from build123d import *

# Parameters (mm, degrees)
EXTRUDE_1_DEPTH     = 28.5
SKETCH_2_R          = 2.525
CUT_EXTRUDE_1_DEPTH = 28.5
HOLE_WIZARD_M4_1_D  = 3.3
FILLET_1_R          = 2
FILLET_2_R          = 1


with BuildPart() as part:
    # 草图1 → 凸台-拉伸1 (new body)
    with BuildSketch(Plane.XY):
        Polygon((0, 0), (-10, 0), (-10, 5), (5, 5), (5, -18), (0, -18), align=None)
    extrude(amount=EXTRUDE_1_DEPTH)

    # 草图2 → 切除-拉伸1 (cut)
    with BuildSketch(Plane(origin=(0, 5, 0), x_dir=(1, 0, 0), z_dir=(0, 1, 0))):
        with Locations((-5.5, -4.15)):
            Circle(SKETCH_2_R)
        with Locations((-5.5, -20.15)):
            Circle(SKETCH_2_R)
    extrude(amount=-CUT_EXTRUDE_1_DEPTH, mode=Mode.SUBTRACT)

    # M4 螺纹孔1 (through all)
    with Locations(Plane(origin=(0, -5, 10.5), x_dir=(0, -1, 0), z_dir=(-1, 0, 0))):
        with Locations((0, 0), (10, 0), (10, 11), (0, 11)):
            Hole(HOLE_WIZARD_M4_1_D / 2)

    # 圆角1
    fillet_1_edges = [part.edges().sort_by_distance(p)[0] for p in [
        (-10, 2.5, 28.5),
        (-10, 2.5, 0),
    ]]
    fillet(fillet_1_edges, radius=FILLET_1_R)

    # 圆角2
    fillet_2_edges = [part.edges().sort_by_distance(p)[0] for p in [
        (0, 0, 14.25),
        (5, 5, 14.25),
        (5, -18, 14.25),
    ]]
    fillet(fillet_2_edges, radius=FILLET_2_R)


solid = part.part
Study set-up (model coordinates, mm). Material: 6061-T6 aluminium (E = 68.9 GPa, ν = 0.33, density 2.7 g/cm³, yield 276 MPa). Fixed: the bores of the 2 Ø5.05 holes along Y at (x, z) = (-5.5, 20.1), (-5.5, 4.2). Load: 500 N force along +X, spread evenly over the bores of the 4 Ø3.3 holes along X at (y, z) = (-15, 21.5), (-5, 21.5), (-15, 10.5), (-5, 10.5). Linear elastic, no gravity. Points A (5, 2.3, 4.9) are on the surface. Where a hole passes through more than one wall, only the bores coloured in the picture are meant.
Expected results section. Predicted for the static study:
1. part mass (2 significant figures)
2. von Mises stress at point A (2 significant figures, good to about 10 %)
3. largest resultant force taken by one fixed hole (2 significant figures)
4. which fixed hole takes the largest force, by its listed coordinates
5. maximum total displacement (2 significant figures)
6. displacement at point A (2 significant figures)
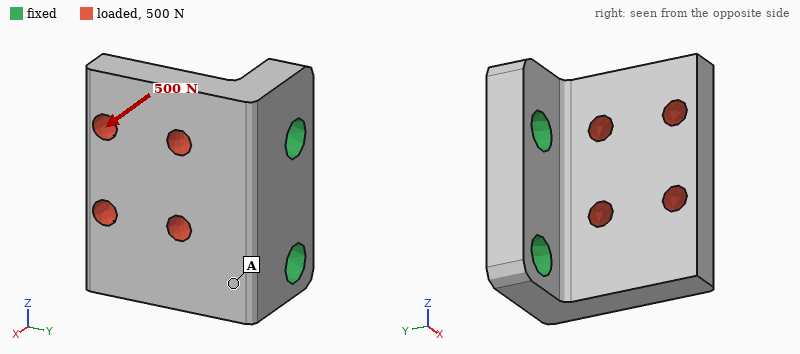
12 g
15 MPa
360 N
(-5.5, 20.1)
70 µm
11 µm
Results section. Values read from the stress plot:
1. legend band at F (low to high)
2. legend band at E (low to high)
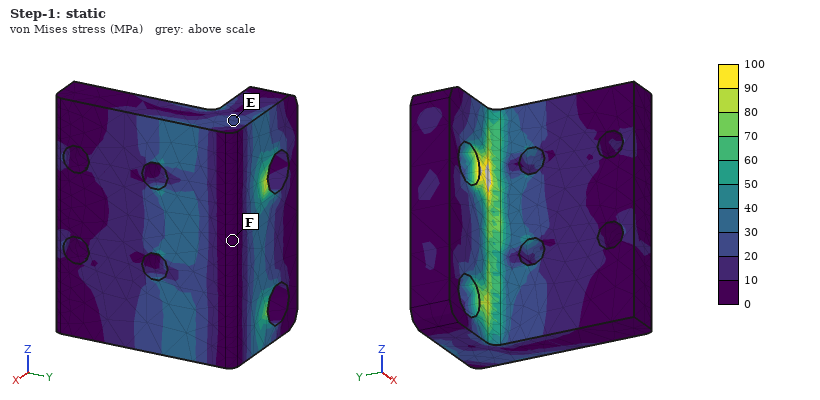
0 to 10 MPa
20 to 30 MPa
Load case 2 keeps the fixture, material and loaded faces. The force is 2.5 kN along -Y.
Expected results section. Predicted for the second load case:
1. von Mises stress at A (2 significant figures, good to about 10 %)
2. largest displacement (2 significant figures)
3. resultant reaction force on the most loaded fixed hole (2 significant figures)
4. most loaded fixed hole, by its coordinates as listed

16 MPa
79 µm
1.7 kN
(-5.5, 20.1)
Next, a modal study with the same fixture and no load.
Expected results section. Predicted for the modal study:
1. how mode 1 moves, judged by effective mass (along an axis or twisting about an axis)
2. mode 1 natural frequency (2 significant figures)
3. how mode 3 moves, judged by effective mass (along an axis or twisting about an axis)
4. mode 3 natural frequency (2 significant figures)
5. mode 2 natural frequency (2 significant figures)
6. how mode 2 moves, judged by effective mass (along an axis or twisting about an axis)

along X
7000 Hz
along Z
17 kHz
13 kHz
along Z
